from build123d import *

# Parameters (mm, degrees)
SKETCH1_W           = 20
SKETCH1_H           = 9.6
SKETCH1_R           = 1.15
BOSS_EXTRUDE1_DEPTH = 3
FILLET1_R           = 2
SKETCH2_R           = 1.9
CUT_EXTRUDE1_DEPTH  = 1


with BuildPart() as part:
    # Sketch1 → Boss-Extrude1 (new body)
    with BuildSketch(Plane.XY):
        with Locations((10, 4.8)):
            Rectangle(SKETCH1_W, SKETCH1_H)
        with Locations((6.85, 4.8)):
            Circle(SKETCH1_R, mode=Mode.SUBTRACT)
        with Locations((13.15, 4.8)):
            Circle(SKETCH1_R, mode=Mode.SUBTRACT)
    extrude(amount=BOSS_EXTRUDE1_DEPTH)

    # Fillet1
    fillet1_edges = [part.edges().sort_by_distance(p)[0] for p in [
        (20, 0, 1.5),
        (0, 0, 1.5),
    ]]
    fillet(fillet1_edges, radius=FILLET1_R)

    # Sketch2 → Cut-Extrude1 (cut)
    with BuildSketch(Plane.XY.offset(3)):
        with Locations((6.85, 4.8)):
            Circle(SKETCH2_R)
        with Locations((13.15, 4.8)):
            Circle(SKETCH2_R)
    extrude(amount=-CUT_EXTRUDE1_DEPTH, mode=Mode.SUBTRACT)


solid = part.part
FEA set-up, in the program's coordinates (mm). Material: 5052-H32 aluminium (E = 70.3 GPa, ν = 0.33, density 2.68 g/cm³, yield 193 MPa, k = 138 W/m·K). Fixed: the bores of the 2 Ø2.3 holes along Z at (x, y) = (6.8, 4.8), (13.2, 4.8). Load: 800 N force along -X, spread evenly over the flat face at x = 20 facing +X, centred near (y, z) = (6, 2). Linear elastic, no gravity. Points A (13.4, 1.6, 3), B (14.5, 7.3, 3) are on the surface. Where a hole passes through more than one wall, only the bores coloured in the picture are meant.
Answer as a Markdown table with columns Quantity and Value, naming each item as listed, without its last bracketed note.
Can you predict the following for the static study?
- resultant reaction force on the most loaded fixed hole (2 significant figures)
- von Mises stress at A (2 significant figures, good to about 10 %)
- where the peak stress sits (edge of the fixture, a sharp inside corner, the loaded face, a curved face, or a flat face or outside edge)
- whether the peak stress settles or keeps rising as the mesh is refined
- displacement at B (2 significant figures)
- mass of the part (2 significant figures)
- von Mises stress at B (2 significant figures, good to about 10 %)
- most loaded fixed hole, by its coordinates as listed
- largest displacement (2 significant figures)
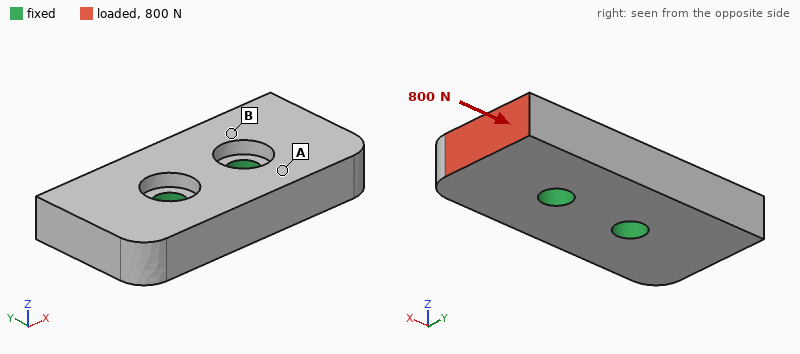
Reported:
| Quantity | Value |
|---|---|
| resultant reaction force on the most loaded fixed hole | 620 N |
| von Mises stress at A | 19 MPa |
| where the peak stress sits | edge of the fixture |
| whether the peak stress settles or keeps rising as the mesh is refined | keeps rising |
| displacement at B | 3.3 µm |
| mass of the part | 1.4 g |
| von Mises stress at B | 44 MPa |
| most loaded fixed hole, by its coordinates as listed | (13.2, 4.8) |
| largest displacement | 8.8 µm |
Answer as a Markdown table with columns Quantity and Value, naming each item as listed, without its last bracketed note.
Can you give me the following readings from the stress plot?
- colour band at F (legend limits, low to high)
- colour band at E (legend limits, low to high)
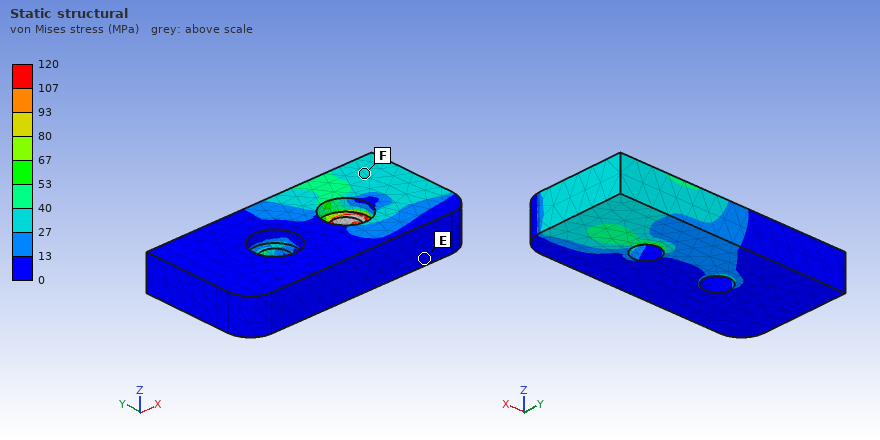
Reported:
| Quantity | Value |
|---|---|
| colour band at F | 27 to 40 MPa |
| colour band at E | 0 to 13 MPa |
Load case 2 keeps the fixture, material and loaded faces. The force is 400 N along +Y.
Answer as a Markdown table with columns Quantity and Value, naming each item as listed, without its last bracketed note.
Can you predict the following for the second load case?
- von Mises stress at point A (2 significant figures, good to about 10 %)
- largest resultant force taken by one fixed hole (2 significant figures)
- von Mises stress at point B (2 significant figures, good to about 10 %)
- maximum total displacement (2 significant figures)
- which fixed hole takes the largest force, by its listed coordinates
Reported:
| Quantity | Value |
|---|---|
| von Mises stress at point A | 28 MPa |
| largest resultant force taken by one fixed hole | 660 N |
| von Mises stress at point B | 23 MPa |
| maximum total displacement | 16 µm |
| which fixed hole takes the largest force, by its listed coordinates | (13.2, 4.8) |
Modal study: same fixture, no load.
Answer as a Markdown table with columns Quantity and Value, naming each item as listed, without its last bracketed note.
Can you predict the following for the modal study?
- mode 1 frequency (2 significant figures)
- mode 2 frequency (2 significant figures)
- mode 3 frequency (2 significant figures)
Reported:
| Quantity | Value |
|---|---|
| mode 1 frequency | 38 kHz |
| mode 2 frequency | 39 kHz |
| mode 3 frequency | 46 kHz |
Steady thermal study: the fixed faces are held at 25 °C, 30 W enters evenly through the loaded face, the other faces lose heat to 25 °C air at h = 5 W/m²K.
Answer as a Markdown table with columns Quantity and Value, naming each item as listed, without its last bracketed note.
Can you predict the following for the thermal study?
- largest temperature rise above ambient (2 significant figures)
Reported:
| Quantity | Value |
|---|---|
| largest temperature rise above ambient | 67 K |
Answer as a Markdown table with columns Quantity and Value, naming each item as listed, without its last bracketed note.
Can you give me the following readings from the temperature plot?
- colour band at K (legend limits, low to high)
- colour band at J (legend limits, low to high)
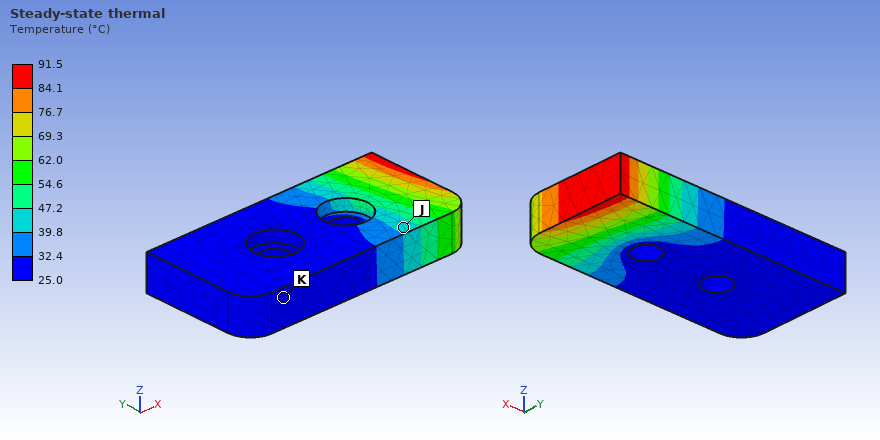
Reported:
| Quantity | Value |
|---|---|
| colour band at K | 25.0 to 32.4 °C |
| colour band at J | 39.8 to 47.2 °C |
